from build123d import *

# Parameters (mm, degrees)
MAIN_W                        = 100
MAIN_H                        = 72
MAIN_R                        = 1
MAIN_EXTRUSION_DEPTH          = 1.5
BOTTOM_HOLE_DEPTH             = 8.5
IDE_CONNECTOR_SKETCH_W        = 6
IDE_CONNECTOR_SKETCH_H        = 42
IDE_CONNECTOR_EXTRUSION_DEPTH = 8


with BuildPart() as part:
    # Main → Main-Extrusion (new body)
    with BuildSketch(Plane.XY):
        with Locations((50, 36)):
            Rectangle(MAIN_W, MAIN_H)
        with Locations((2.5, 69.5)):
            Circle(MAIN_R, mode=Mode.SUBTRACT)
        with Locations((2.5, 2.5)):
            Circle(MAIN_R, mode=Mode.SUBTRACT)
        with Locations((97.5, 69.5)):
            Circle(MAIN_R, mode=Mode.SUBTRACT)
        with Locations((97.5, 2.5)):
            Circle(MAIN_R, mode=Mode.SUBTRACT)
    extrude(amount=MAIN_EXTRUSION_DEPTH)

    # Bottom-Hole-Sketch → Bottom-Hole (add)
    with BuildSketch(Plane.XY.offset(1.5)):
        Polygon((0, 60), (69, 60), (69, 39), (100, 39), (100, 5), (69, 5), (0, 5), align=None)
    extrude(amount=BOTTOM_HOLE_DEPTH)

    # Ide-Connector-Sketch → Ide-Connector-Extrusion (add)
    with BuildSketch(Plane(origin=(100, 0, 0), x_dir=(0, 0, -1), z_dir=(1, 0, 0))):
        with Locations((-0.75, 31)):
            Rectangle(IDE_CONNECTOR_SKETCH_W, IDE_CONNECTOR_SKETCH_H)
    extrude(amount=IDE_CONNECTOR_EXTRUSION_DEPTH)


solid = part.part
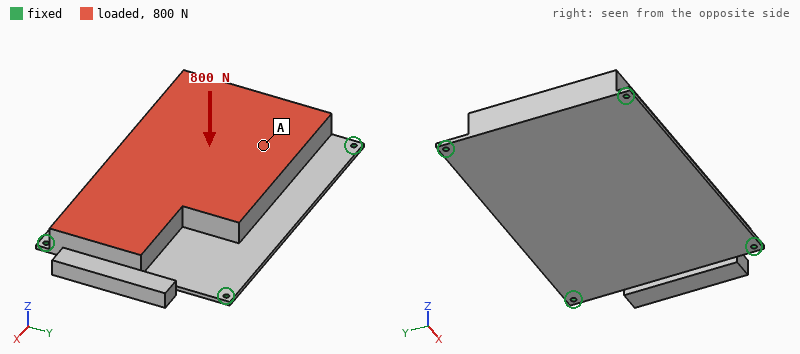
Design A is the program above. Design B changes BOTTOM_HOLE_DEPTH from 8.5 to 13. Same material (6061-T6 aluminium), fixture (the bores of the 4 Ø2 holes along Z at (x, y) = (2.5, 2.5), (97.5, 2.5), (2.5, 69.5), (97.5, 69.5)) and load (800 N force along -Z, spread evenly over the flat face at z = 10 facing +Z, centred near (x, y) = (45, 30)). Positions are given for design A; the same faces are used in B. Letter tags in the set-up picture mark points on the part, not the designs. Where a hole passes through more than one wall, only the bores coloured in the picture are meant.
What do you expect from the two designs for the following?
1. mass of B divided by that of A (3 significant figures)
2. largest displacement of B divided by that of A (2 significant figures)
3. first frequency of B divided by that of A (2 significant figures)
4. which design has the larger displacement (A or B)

1.40
0.84
0.91
A
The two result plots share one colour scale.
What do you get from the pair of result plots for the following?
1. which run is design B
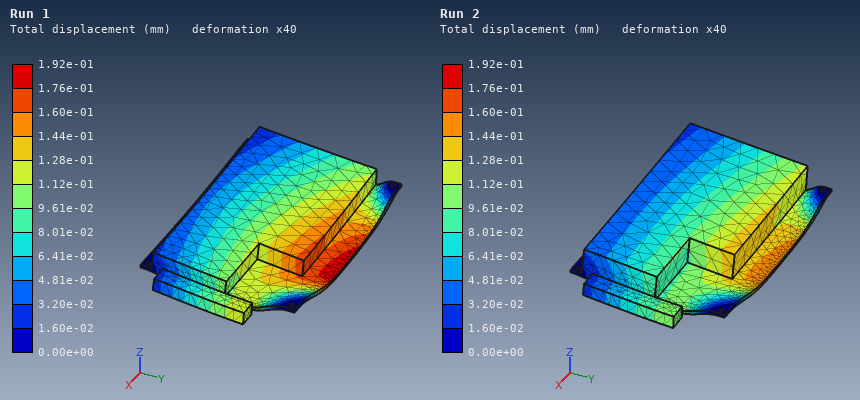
Run 2
